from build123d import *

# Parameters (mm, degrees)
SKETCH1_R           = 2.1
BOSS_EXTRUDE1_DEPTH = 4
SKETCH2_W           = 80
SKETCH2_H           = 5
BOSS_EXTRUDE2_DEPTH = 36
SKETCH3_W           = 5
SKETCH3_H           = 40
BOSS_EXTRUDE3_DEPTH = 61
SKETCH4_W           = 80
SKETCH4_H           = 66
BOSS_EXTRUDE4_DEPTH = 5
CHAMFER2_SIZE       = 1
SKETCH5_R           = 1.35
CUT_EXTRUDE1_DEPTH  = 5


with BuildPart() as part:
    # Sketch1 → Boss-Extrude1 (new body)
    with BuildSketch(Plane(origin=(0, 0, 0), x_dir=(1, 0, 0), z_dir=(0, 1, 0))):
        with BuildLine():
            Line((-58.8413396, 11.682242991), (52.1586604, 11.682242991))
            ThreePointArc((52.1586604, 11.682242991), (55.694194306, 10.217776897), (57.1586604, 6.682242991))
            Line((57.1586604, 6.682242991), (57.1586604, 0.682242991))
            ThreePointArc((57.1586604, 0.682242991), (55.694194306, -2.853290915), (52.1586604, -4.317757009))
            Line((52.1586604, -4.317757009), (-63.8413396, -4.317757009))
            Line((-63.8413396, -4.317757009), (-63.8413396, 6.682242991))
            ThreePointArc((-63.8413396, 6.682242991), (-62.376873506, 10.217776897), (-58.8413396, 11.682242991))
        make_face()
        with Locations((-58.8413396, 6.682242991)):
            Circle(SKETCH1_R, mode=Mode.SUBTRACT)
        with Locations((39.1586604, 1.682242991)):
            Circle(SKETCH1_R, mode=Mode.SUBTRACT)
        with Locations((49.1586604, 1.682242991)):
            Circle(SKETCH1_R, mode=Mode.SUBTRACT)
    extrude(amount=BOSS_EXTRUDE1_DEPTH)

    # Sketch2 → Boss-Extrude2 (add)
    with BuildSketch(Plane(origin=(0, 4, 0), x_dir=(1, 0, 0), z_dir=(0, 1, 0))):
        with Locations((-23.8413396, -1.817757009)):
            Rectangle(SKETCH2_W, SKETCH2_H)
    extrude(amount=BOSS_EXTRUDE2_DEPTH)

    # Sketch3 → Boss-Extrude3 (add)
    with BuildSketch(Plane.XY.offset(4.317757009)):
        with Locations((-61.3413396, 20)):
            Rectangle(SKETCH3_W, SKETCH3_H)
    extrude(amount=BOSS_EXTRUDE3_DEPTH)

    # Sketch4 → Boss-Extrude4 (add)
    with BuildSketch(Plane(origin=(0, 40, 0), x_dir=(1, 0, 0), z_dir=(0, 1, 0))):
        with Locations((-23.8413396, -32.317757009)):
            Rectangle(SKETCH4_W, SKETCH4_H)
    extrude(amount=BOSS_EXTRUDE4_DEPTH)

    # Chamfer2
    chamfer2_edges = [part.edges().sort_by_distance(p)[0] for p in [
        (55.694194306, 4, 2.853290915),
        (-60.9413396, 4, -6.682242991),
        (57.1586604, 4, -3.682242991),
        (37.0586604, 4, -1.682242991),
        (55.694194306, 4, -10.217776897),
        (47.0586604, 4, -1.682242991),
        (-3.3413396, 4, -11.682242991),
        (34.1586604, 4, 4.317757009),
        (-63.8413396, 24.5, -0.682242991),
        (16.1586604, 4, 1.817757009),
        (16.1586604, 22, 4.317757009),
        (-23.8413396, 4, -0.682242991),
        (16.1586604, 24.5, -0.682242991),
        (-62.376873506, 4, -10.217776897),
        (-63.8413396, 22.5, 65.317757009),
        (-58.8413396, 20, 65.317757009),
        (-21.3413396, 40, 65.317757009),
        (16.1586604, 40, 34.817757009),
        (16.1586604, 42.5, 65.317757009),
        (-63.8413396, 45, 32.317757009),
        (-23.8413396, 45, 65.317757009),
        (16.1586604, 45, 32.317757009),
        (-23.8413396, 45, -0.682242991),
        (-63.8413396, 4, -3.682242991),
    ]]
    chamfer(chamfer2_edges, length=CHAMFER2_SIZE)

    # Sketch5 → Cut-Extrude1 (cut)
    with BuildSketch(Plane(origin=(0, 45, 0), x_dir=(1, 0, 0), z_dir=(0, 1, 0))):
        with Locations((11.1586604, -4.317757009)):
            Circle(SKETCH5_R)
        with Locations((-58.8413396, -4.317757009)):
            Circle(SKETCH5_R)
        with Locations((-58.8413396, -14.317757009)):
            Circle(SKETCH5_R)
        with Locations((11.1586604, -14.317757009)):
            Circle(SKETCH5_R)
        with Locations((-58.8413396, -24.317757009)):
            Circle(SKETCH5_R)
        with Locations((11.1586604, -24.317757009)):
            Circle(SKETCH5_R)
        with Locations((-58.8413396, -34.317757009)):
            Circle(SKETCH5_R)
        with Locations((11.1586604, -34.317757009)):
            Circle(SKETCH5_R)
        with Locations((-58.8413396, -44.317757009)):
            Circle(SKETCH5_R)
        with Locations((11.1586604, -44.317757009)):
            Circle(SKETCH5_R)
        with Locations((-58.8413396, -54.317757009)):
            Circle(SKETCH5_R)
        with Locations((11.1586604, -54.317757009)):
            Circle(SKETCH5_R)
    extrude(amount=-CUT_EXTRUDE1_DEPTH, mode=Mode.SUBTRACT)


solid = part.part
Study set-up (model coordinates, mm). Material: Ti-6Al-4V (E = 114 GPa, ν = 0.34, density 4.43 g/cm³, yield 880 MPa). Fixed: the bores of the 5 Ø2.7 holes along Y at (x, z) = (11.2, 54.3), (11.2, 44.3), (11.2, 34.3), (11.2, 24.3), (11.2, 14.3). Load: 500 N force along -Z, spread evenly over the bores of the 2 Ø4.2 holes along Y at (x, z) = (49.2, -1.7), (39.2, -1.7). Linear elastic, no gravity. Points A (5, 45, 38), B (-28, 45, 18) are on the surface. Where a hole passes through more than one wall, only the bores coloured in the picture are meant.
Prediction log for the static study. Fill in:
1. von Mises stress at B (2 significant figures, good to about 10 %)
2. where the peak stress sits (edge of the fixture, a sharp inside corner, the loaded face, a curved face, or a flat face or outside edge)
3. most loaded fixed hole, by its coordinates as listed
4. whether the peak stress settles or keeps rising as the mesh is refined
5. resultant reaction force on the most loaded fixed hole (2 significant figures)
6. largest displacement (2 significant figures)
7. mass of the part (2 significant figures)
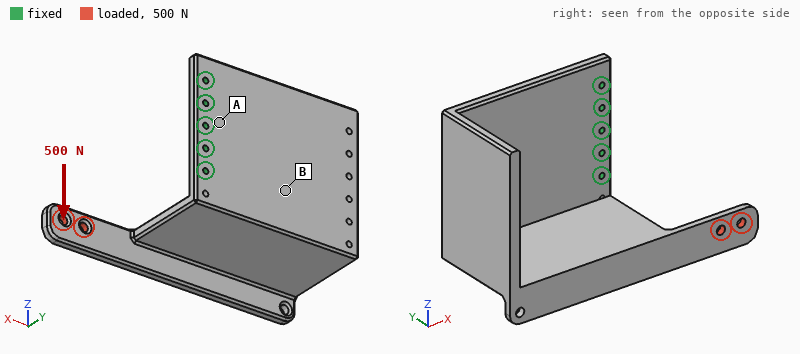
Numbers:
27 MPa
edge of the fixture
(11.2, 14.3)
keeps rising
900 N
0.92 mm
260 g
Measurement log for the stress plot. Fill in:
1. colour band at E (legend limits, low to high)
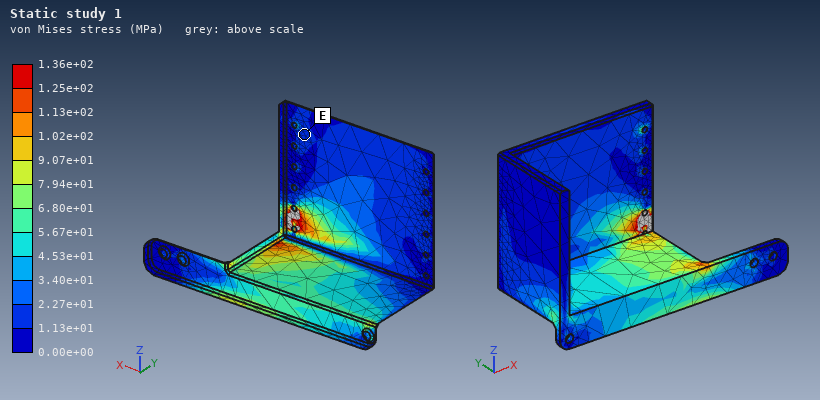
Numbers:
1.13e+01 to 2.27e+01 MPa
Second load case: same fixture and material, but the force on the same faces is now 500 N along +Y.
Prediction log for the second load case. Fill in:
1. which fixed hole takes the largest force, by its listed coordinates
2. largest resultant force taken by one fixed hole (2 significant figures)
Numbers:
(11.2, 14.3)
870 N
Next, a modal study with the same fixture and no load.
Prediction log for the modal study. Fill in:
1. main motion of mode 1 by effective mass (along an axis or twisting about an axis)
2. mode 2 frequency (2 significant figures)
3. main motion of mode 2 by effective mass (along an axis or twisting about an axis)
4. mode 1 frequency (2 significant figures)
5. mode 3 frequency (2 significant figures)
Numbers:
along Y
720 Hz
along Z
430 Hz
1200 Hz
